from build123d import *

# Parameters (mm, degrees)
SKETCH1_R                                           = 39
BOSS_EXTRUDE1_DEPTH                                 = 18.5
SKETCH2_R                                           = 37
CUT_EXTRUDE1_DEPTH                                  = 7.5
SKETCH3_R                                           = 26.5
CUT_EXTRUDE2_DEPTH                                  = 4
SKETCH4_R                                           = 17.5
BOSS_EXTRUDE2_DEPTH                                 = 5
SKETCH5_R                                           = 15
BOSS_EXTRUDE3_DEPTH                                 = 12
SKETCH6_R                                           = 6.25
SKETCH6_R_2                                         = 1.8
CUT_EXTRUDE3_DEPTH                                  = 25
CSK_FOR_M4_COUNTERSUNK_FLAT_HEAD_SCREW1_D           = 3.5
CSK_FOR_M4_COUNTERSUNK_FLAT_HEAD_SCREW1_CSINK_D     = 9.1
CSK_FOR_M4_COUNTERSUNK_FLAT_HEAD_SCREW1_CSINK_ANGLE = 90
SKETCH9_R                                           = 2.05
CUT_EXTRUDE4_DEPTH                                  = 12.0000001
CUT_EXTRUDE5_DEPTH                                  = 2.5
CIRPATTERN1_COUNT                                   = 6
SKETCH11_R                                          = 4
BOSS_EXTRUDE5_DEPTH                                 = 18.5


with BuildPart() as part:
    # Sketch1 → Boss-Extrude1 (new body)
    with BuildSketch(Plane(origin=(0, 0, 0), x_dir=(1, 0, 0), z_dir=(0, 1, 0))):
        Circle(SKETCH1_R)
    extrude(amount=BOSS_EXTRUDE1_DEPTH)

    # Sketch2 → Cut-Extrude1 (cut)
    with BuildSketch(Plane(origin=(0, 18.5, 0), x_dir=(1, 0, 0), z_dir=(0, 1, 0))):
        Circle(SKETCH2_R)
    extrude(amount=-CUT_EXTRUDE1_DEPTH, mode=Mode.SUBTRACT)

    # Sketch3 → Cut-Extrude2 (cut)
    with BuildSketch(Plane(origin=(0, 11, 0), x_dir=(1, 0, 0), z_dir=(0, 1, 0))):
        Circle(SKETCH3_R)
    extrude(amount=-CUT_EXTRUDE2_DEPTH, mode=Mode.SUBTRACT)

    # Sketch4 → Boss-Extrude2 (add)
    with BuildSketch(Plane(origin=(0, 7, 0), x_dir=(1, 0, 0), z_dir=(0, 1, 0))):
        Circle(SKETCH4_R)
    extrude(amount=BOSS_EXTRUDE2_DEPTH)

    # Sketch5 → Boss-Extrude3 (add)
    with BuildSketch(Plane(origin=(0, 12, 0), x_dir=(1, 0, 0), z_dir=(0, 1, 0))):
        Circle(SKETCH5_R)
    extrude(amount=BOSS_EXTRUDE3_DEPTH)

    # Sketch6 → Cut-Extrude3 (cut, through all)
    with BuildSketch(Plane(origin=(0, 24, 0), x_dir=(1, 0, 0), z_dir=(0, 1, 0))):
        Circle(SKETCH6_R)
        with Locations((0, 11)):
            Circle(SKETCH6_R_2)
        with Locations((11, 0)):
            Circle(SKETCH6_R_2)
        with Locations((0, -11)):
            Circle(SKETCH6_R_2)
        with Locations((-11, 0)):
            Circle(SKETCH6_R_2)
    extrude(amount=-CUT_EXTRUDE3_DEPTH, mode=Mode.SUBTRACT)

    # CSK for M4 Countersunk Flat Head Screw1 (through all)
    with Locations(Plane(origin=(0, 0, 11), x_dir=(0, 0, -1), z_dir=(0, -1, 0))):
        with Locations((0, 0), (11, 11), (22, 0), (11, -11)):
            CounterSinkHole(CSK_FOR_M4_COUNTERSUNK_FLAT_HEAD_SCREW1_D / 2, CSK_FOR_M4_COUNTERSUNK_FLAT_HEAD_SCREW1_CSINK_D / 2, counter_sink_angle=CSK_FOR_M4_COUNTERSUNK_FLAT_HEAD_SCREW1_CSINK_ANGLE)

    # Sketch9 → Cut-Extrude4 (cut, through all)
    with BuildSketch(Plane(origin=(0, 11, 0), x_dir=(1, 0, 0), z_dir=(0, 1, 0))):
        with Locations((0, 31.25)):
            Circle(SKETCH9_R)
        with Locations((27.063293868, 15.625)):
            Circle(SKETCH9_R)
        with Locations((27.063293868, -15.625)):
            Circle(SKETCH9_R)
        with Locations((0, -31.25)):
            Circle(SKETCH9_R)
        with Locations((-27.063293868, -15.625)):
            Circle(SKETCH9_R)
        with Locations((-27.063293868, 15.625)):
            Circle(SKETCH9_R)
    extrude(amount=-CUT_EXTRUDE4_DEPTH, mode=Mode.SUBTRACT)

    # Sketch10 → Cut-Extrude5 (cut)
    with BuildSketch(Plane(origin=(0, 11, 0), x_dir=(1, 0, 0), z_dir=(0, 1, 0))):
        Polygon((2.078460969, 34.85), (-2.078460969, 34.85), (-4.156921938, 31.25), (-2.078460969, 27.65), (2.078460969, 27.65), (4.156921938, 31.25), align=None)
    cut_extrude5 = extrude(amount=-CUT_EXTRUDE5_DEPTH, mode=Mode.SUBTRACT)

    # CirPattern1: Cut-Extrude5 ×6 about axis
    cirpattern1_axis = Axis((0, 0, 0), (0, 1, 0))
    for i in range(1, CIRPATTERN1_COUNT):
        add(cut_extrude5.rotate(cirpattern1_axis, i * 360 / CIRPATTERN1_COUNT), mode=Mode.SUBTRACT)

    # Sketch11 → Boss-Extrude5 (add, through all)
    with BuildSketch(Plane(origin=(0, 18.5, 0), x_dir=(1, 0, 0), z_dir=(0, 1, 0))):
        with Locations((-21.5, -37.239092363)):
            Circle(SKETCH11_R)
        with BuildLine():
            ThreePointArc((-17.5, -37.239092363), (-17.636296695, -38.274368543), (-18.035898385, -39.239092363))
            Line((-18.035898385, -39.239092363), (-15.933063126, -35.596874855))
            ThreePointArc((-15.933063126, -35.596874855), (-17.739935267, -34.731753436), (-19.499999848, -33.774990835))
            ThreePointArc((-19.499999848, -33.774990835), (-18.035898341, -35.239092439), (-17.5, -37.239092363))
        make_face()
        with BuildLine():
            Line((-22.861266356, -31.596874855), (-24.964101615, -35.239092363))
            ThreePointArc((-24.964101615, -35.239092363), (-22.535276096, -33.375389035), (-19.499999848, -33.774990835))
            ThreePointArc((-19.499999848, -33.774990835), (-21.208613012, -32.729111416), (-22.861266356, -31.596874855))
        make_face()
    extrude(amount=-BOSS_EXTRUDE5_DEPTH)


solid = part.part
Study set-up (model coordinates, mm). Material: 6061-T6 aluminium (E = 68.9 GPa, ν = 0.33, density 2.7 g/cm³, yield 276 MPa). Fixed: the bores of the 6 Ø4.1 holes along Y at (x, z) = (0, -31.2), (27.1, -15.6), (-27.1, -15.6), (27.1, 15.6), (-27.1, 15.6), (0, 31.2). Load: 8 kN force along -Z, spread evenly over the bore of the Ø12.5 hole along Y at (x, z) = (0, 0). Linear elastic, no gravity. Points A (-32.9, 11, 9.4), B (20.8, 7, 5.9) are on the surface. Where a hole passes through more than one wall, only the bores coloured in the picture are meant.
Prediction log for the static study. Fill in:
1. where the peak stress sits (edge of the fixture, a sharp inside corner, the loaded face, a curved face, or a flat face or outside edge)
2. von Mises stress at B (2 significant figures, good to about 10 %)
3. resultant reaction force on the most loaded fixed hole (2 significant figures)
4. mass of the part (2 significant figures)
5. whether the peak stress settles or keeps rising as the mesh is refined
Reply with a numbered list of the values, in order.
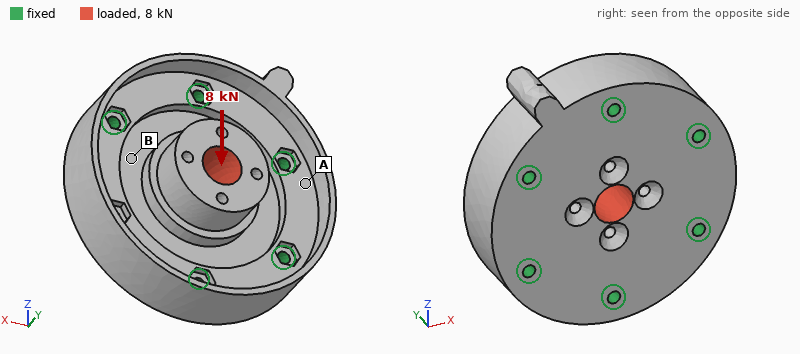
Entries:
1. edge of the fixture
2. 18 MPa
3. 2.2 kN
4. 150 g
5. keeps rising
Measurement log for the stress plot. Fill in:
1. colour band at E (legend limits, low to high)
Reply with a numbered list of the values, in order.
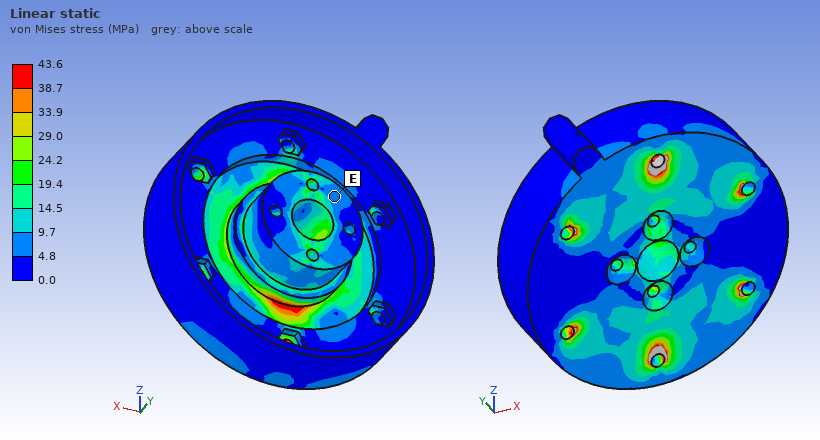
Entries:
1. 4.8 to 9.7 MPa
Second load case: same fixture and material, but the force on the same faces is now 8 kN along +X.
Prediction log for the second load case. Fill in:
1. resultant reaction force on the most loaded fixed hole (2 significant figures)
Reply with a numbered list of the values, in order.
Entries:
1. 1.9 kN
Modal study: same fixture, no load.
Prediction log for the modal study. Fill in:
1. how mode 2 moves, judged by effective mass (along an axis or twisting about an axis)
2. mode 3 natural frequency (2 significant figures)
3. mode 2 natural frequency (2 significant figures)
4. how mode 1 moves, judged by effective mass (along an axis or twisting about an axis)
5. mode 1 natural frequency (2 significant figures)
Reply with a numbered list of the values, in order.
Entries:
1. along Y
2. 17 kHz
3. 15 kHz
4. along Y
5. 14 kHz
